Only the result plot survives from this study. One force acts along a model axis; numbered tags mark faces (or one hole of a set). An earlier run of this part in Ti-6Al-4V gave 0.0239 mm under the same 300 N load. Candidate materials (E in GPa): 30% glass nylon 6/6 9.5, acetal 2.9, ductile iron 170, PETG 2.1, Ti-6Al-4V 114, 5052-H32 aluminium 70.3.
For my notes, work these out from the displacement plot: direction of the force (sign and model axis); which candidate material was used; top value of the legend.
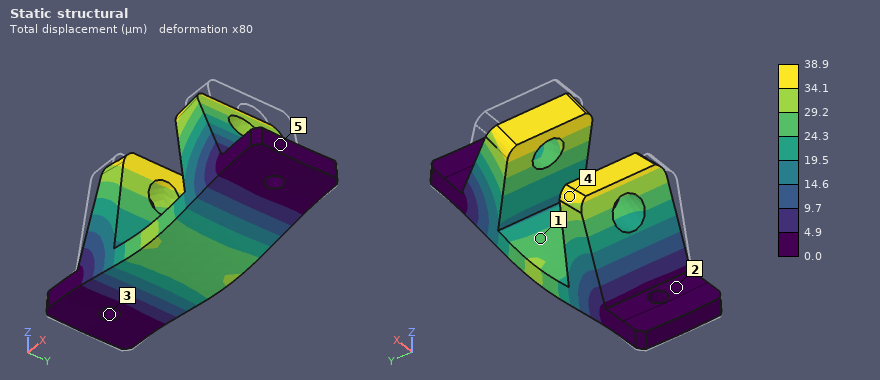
-Z
5052-H32 aluminium
38.9 µm
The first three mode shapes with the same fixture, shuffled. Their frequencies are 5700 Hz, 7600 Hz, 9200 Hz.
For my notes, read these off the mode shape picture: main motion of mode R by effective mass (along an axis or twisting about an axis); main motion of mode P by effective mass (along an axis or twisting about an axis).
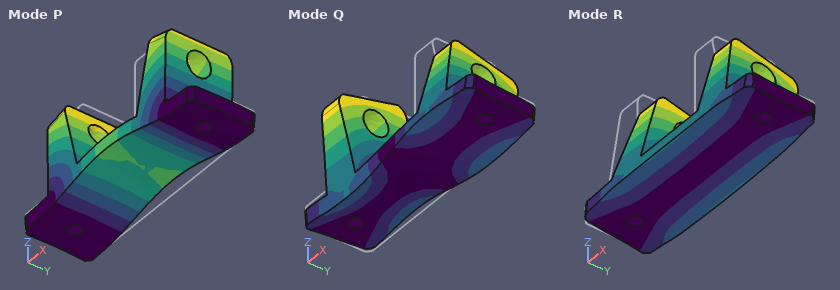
along Y
along Z
